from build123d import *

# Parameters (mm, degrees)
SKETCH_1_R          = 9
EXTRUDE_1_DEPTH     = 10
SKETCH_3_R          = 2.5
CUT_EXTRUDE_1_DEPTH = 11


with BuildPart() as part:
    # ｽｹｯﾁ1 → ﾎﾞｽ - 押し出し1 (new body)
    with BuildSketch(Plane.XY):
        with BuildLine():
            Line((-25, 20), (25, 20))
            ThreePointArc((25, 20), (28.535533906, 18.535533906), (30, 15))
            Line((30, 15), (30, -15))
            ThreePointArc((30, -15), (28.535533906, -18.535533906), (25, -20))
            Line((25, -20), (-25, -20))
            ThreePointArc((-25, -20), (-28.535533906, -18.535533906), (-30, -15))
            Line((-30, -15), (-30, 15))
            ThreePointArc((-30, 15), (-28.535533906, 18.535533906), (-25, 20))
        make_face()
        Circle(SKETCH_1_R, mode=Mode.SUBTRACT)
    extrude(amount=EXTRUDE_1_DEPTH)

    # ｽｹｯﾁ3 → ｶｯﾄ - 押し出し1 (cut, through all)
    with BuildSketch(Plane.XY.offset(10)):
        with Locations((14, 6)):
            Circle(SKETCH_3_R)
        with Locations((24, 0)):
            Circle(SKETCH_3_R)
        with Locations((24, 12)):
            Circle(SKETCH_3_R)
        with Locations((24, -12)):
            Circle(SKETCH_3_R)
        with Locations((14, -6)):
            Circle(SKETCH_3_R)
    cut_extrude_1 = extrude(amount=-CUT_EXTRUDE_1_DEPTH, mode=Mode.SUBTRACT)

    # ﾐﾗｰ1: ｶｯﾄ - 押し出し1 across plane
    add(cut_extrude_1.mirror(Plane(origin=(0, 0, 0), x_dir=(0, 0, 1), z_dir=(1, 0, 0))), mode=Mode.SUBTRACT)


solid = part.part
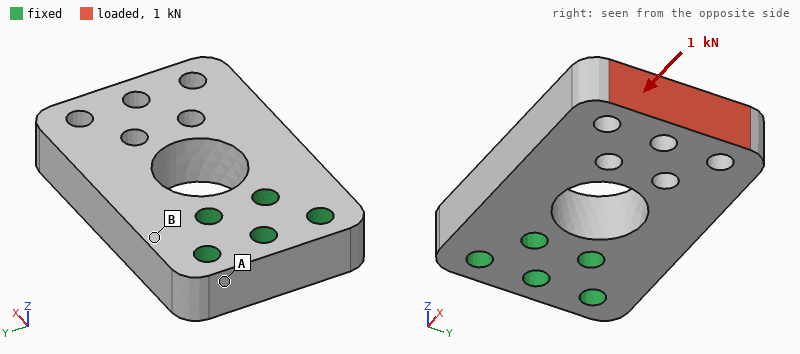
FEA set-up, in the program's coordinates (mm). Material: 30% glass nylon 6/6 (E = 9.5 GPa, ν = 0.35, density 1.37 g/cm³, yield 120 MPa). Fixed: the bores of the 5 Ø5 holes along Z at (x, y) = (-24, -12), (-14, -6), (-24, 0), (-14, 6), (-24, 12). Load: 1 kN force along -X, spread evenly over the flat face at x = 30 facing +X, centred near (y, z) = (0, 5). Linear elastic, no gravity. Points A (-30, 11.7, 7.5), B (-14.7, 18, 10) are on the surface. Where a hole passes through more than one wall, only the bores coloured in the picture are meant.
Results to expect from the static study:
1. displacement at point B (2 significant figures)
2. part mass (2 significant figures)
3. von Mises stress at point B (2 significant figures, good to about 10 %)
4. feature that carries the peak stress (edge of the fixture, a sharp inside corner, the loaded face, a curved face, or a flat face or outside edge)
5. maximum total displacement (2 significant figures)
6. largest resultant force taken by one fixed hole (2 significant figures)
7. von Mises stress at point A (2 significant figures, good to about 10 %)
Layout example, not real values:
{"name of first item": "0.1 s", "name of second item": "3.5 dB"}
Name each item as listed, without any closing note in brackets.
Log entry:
{"displacement at point B": "4.7 µm", "part mass": "26 g", "von Mises stress at point B": "3.6 MPa", "feature that carries the peak stress": "a curved face", "maximum total displacement": "29 µm", "largest resultant force taken by one fixed hole": "290 N", "von Mises stress at point A": "1.3 MPa"}
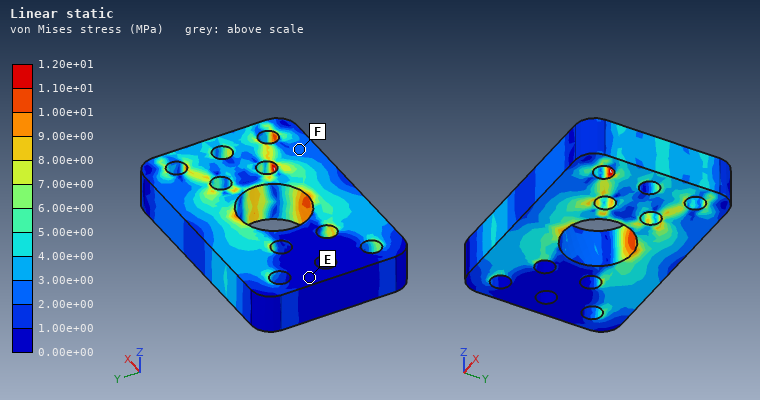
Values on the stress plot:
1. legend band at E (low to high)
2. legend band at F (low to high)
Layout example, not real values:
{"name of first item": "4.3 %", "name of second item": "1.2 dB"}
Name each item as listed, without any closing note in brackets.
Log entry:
{"legend band at E": "0.00e+00 to 1.00e+00 MPa", "legend band at F": "2.00e+00 to 3.00e+00 MPa"}
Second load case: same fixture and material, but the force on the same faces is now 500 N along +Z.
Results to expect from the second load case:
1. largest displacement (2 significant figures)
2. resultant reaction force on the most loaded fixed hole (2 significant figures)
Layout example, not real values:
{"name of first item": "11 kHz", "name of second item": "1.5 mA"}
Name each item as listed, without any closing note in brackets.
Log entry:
{"largest displacement": "0.80 mm", "resultant reaction force on the most loaded fixed hole": "550 N"}
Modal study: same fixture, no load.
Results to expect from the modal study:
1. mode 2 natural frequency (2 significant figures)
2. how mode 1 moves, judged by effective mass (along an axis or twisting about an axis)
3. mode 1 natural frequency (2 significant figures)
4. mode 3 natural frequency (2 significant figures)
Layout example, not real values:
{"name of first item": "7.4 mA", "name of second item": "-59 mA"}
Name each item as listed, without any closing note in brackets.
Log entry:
{"mode 2 natural frequency": "4000 Hz", "how mode 1 moves, judged by effective mass": "along Z", "mode 1 natural frequency": "1800 Hz", "mode 3 natural frequency": "4100 Hz"}
